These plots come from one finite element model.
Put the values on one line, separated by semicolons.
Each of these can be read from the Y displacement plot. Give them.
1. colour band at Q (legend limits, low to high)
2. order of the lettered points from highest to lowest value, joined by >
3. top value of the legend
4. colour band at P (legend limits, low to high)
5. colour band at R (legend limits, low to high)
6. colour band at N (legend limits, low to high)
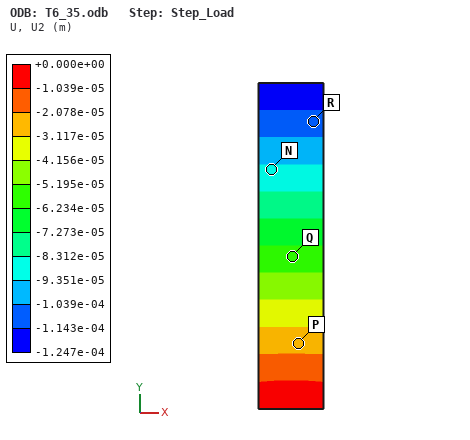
-6.234e-05 to -5.195e-05 m; P > Q > N > R; +0.000e+00 m; -3.117e-05 to -2.078e-05 m; -1.143e-04 to -1.039e-04 m; -9.351e-05 to -8.312e-05 m
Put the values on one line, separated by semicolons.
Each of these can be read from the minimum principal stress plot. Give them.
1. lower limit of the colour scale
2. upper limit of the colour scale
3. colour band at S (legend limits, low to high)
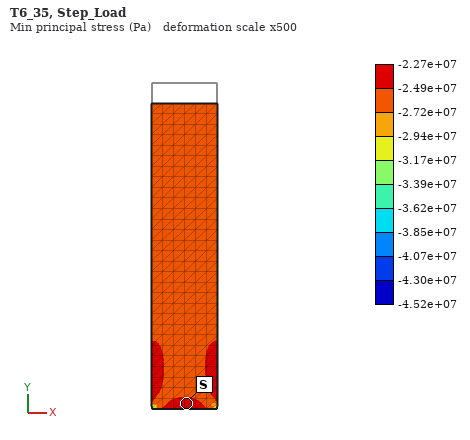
-4.52e+07 Pa; -2.27e+07 Pa; -2.49e+07 to -2.27e+07 Pa
